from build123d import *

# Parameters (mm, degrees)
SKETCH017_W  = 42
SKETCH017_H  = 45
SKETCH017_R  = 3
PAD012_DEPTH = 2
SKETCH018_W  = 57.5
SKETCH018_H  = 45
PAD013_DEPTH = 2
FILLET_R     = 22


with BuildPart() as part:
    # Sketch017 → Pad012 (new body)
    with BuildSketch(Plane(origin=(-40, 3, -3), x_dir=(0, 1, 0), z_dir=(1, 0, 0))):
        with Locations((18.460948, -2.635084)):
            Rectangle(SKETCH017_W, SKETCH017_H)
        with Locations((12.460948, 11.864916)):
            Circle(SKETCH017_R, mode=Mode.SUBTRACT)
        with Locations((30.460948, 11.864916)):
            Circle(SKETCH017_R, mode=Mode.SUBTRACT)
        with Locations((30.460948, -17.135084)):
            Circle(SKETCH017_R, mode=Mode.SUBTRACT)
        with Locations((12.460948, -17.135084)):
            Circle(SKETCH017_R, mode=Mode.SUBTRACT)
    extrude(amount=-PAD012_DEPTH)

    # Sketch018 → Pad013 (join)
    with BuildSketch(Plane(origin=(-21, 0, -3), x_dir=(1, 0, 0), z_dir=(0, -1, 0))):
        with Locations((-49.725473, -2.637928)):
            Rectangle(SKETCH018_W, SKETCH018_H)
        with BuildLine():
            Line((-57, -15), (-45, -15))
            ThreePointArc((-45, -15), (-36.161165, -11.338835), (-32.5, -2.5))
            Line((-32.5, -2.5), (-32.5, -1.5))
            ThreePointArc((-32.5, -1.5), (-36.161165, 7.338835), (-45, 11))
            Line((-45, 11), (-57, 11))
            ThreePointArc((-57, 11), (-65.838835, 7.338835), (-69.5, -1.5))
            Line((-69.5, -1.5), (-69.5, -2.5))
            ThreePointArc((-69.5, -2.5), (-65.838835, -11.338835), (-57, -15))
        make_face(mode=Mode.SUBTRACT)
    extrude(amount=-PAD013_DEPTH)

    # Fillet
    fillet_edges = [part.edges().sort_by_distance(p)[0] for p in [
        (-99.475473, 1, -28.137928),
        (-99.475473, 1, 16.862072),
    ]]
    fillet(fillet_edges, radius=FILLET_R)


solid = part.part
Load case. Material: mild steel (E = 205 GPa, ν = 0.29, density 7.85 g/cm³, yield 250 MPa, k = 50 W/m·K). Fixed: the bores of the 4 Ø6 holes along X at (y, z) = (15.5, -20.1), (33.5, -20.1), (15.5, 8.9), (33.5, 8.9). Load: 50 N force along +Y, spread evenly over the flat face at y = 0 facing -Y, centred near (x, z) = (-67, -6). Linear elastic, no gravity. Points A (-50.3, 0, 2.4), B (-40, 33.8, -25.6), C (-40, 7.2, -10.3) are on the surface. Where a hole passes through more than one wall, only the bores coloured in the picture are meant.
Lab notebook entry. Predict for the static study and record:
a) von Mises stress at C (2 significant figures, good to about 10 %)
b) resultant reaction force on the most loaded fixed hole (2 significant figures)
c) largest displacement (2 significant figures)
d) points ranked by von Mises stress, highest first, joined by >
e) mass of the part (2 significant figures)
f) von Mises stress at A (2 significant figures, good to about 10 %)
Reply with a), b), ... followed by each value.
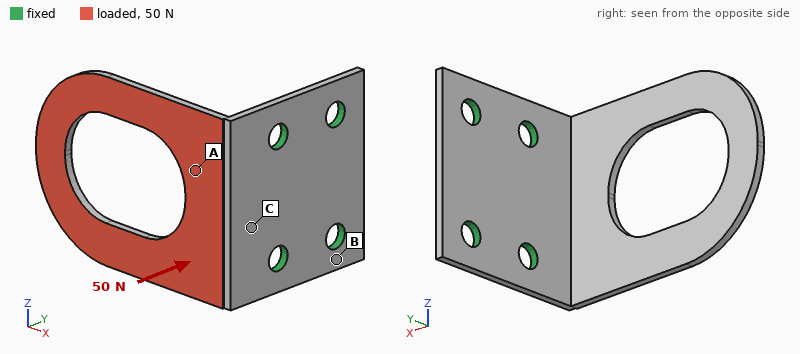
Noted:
a) 34 MPa
b) 22 N
c) 0.41 mm
d) C > A > B
e) 52 g
f) 27 MPa
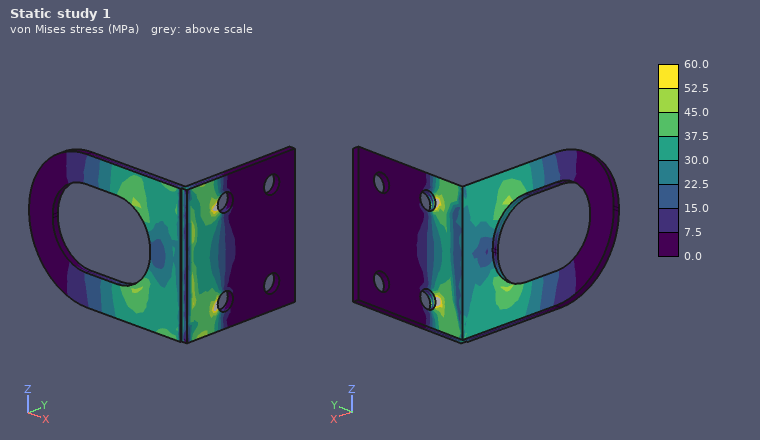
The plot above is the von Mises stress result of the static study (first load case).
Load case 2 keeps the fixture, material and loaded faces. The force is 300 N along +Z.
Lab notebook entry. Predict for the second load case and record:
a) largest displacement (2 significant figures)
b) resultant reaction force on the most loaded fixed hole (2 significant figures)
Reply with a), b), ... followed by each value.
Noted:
a) 0.15 mm
b) 310 N
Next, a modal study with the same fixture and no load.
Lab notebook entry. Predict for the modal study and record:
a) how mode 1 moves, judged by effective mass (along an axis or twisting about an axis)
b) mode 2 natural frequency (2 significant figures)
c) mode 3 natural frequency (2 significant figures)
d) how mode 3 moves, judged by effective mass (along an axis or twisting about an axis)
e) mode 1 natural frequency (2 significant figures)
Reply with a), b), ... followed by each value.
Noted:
a) along Y
b) 1300 Hz
c) 1800 Hz
d) along Z
e) 440 Hz
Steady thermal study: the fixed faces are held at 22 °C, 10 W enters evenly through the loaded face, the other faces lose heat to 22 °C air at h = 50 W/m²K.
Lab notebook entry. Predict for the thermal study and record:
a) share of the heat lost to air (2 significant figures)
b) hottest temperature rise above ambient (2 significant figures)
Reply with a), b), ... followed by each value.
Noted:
a) 50 %
b) 61 K
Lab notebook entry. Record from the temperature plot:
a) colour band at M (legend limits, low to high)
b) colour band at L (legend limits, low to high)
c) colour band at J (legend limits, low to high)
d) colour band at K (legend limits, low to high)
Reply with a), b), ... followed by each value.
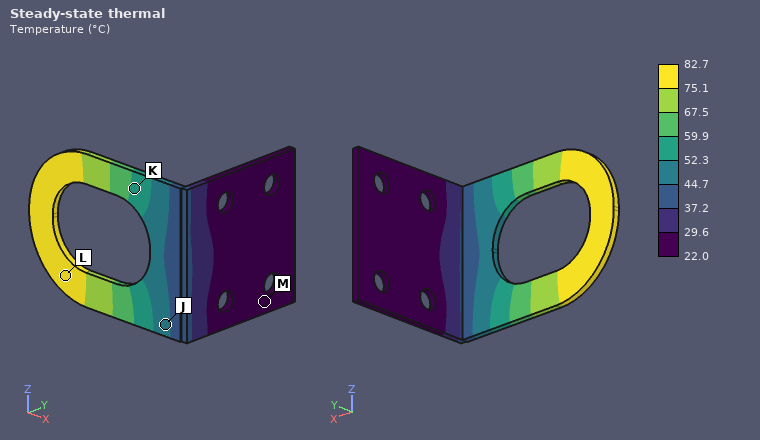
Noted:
a) 22.0 to 29.6 °C
b) 75.1 to 82.7 °C
c) 44.7 to 52.3 °C
d) 52.3 to 59.9 °C
